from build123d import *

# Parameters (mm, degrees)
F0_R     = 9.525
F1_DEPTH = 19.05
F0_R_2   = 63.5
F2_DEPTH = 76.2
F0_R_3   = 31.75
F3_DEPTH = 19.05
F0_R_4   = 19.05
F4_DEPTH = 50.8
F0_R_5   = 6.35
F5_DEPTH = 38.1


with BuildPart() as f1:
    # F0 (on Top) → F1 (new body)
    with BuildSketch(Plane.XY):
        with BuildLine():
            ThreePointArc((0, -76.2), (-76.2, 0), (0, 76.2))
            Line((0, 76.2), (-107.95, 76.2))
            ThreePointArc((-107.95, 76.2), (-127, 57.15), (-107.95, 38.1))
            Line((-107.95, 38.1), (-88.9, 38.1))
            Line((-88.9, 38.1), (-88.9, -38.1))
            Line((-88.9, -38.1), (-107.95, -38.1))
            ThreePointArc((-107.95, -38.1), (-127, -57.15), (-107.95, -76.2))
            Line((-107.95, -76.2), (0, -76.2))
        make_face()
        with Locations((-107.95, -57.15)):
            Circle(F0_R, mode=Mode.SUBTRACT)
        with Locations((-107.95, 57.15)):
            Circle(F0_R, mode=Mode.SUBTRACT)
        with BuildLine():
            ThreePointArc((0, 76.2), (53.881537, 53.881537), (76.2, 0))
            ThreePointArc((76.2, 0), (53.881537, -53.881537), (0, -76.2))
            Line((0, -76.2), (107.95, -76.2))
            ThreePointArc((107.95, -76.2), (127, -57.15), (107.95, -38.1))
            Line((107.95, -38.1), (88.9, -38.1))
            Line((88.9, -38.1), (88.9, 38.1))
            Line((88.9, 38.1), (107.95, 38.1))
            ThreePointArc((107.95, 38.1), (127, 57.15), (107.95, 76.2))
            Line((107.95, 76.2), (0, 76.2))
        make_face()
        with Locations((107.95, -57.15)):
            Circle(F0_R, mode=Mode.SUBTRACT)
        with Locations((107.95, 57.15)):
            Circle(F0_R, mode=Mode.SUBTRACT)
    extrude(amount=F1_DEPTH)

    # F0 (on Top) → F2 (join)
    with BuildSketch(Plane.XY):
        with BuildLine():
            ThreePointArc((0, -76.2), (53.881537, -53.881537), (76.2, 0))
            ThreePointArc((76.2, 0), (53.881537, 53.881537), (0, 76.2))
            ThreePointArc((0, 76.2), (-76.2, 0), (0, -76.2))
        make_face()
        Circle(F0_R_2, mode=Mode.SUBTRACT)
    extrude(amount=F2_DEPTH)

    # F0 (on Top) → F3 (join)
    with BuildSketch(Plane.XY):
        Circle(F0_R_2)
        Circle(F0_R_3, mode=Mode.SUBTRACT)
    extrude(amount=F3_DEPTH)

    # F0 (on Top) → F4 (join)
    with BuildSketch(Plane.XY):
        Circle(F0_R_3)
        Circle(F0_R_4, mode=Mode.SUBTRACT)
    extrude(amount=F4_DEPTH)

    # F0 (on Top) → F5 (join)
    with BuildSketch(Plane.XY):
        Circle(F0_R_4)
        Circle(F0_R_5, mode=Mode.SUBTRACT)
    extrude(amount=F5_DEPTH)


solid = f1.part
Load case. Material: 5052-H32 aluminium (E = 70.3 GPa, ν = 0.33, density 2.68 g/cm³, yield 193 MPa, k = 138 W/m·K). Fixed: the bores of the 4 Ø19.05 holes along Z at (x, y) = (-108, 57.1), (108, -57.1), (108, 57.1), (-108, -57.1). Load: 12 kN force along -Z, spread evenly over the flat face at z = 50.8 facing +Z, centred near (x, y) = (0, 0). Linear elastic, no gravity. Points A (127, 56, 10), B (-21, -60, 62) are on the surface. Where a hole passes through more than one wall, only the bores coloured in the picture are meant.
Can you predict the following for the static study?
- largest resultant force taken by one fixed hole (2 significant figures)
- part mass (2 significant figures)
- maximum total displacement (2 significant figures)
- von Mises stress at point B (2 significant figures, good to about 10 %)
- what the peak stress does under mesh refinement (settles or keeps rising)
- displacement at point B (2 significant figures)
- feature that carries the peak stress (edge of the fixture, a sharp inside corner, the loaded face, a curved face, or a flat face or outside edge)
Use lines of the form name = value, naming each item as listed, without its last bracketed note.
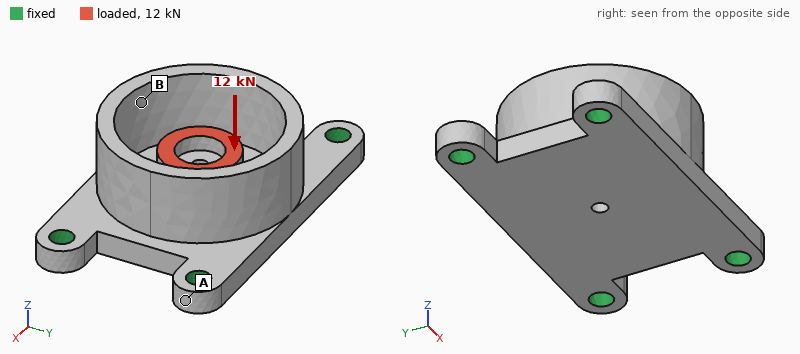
largest resultant force taken by one fixed hole = 3.3 kN
part mass = 2.7 kg
maximum total displacement = 63 µm
von Mises stress at point B = 7.2 MPa
what the peak stress does under mesh refinement = keeps rising
displacement at point B = 44 µm
feature that carries the peak stress = edge of the fixture
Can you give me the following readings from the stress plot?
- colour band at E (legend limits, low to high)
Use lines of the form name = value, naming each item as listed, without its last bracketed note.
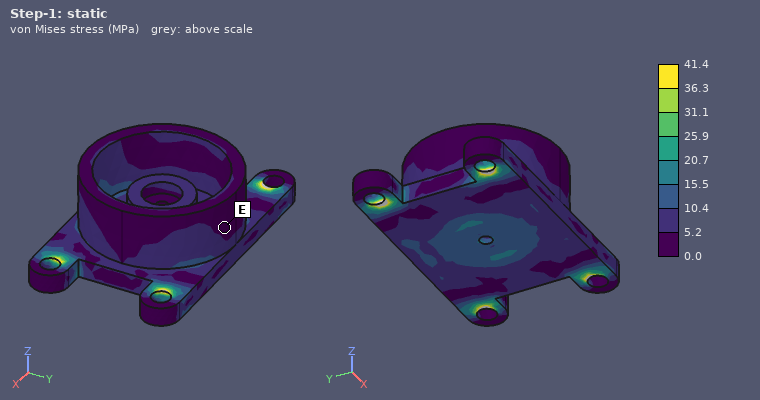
colour band at E = 0.0 to 5.2 MPa
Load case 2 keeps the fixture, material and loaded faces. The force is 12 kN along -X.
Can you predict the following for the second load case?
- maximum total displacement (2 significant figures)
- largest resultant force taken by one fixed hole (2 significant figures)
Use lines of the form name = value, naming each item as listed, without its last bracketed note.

maximum total displacement = 55 µm
largest resultant force taken by one fixed hole = 3.5 kN
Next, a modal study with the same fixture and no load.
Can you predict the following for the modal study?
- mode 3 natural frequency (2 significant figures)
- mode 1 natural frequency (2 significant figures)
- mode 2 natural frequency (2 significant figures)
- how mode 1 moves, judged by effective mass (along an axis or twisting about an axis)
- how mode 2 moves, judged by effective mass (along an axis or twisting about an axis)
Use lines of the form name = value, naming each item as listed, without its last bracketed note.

mode 3 natural frequency = 3500 Hz
mode 1 natural frequency = 1800 Hz
mode 2 natural frequency = 2200 Hz
how mode 1 moves, judged by effective mass = along Z
how mode 2 moves, judged by effective mass = along Y
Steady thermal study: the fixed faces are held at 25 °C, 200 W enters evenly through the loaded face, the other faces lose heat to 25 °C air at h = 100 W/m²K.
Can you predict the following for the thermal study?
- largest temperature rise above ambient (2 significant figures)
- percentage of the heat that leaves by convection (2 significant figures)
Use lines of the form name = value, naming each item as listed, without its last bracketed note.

largest temperature rise above ambient = 38 K
percentage of the heat that leaves by convection = 60 %
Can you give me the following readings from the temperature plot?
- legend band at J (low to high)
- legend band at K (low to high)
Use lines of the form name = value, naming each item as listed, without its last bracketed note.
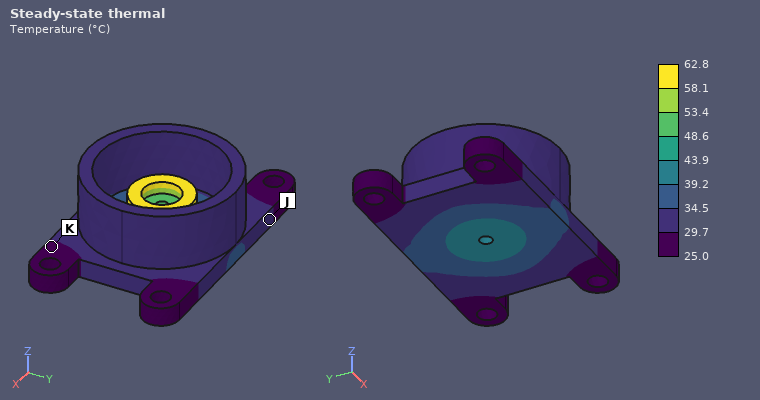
legend band at J = 29.7 to 34.5 °C
legend band at K = 25.0 to 29.7 °C
